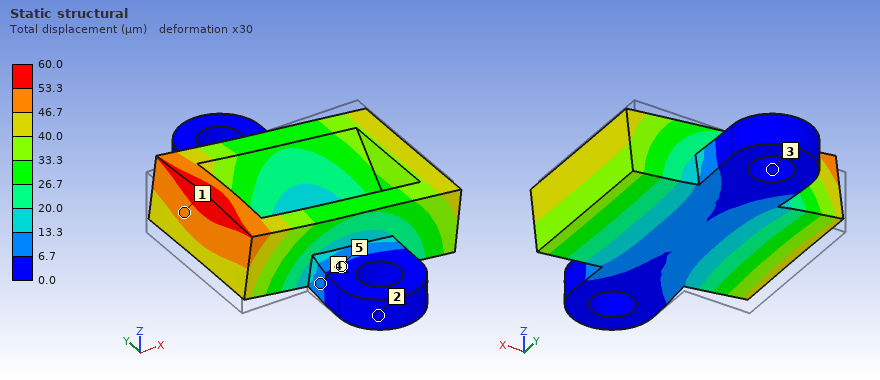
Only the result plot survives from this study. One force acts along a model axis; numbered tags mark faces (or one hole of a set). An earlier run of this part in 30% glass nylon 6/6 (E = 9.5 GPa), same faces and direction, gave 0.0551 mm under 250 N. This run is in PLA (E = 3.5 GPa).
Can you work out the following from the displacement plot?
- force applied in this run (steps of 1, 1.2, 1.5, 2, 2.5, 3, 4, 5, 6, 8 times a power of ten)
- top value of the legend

100 N
60.0 µm
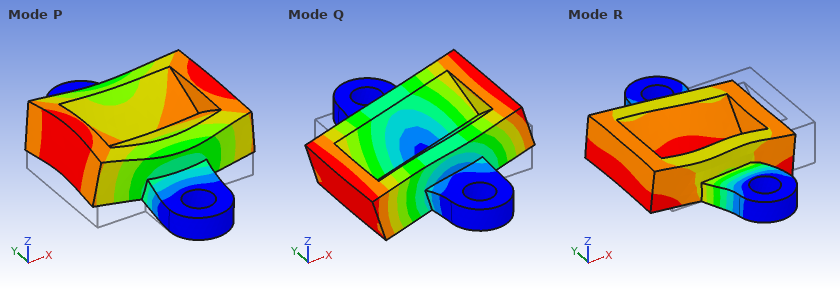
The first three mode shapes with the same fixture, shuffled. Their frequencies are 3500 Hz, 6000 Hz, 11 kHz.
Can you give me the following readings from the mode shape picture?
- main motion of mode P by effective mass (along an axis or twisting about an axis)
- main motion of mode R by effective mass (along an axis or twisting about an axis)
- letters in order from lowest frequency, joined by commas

along Z
along X
Q, P, R
